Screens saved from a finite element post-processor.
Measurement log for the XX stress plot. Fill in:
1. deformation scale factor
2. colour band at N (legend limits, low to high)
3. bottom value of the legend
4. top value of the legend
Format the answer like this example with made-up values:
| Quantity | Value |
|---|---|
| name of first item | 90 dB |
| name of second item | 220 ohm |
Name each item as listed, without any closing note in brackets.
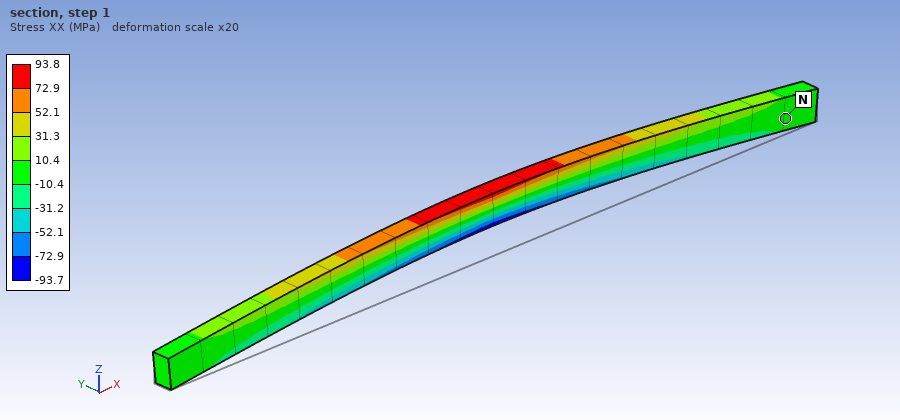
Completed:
| Quantity | Value |
|---|---|
| deformation scale factor | 20 |
| colour band at N | -10.4 to 10.4 MPa |
| bottom value of the legend | -93.7 MPa |
| top value of the legend | 93.8 MPa |
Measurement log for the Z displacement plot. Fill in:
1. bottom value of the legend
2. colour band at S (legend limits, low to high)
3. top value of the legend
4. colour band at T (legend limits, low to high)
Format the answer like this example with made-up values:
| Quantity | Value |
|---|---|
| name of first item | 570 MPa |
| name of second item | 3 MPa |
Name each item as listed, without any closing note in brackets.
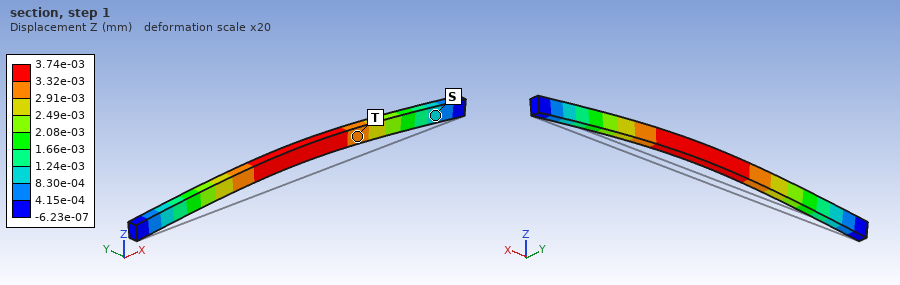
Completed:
| Quantity | Value |
|---|---|
| bottom value of the legend | -6.23e-07 mm |
| colour band at S | 8.30e-04 to 1.24e-03 mm |
| top value of the legend | 3.74e-03 mm |
| colour band at T | 2.91e-03 to 3.32e-03 mm |
